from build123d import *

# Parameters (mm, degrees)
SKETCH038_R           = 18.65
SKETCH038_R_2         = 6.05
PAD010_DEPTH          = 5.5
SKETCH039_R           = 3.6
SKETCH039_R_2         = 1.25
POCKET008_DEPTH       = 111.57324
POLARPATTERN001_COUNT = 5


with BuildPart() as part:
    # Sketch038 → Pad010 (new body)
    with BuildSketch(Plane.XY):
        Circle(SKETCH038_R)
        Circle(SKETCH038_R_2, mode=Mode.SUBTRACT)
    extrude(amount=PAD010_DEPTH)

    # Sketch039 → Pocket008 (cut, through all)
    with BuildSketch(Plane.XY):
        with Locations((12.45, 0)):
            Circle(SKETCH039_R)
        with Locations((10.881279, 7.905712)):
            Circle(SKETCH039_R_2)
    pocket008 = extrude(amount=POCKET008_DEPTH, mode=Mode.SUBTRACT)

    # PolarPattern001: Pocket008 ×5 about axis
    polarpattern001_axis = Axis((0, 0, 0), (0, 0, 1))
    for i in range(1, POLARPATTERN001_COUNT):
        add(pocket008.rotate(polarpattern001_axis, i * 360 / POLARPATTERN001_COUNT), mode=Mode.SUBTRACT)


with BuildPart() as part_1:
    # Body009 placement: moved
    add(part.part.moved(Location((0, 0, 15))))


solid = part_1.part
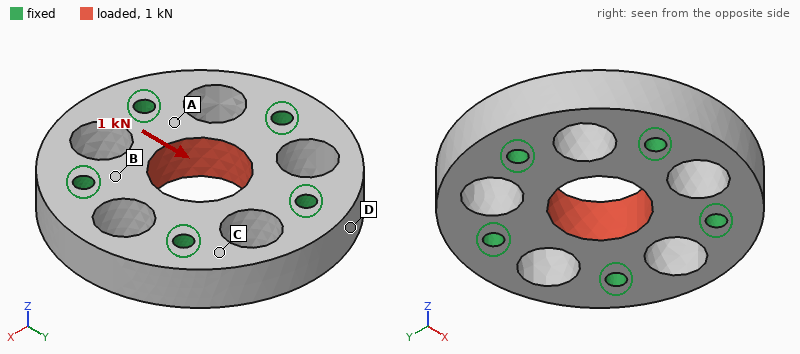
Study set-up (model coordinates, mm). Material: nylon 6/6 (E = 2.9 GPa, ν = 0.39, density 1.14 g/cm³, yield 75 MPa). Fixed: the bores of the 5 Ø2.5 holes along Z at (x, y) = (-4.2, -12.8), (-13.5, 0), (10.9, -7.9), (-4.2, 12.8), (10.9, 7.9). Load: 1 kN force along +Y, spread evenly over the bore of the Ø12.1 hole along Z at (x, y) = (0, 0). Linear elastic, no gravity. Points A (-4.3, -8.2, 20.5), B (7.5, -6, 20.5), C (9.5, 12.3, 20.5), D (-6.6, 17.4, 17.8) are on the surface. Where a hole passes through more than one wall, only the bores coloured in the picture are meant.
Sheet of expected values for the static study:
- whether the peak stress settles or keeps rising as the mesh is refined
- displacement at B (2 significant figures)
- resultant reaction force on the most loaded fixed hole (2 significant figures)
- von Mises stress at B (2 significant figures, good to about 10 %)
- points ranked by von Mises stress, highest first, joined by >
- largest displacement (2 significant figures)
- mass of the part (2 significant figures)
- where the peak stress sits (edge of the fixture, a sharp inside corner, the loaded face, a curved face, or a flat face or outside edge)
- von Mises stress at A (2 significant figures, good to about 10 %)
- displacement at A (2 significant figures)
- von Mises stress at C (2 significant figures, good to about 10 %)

keeps rising
11 µm
290 N
4.8 MPa
A > B > C > D
29 µm
4.7 g
edge of the fixture
6.1 MPa
9.8 µm
2.5 MPa
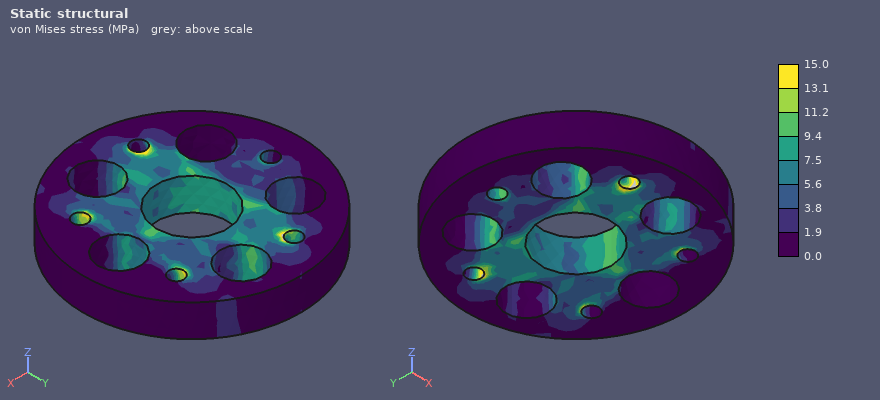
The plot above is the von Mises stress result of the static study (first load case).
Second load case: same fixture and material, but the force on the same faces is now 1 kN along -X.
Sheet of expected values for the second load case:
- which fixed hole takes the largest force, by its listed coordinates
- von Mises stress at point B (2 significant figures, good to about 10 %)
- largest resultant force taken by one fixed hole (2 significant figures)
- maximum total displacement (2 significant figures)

(-13.5, 0)
5.9 MPa
300 N
30 µm
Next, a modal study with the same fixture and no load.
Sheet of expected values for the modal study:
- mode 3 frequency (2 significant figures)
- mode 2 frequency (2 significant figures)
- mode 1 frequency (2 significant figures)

17 kHz
16 kHz
16 kHz
